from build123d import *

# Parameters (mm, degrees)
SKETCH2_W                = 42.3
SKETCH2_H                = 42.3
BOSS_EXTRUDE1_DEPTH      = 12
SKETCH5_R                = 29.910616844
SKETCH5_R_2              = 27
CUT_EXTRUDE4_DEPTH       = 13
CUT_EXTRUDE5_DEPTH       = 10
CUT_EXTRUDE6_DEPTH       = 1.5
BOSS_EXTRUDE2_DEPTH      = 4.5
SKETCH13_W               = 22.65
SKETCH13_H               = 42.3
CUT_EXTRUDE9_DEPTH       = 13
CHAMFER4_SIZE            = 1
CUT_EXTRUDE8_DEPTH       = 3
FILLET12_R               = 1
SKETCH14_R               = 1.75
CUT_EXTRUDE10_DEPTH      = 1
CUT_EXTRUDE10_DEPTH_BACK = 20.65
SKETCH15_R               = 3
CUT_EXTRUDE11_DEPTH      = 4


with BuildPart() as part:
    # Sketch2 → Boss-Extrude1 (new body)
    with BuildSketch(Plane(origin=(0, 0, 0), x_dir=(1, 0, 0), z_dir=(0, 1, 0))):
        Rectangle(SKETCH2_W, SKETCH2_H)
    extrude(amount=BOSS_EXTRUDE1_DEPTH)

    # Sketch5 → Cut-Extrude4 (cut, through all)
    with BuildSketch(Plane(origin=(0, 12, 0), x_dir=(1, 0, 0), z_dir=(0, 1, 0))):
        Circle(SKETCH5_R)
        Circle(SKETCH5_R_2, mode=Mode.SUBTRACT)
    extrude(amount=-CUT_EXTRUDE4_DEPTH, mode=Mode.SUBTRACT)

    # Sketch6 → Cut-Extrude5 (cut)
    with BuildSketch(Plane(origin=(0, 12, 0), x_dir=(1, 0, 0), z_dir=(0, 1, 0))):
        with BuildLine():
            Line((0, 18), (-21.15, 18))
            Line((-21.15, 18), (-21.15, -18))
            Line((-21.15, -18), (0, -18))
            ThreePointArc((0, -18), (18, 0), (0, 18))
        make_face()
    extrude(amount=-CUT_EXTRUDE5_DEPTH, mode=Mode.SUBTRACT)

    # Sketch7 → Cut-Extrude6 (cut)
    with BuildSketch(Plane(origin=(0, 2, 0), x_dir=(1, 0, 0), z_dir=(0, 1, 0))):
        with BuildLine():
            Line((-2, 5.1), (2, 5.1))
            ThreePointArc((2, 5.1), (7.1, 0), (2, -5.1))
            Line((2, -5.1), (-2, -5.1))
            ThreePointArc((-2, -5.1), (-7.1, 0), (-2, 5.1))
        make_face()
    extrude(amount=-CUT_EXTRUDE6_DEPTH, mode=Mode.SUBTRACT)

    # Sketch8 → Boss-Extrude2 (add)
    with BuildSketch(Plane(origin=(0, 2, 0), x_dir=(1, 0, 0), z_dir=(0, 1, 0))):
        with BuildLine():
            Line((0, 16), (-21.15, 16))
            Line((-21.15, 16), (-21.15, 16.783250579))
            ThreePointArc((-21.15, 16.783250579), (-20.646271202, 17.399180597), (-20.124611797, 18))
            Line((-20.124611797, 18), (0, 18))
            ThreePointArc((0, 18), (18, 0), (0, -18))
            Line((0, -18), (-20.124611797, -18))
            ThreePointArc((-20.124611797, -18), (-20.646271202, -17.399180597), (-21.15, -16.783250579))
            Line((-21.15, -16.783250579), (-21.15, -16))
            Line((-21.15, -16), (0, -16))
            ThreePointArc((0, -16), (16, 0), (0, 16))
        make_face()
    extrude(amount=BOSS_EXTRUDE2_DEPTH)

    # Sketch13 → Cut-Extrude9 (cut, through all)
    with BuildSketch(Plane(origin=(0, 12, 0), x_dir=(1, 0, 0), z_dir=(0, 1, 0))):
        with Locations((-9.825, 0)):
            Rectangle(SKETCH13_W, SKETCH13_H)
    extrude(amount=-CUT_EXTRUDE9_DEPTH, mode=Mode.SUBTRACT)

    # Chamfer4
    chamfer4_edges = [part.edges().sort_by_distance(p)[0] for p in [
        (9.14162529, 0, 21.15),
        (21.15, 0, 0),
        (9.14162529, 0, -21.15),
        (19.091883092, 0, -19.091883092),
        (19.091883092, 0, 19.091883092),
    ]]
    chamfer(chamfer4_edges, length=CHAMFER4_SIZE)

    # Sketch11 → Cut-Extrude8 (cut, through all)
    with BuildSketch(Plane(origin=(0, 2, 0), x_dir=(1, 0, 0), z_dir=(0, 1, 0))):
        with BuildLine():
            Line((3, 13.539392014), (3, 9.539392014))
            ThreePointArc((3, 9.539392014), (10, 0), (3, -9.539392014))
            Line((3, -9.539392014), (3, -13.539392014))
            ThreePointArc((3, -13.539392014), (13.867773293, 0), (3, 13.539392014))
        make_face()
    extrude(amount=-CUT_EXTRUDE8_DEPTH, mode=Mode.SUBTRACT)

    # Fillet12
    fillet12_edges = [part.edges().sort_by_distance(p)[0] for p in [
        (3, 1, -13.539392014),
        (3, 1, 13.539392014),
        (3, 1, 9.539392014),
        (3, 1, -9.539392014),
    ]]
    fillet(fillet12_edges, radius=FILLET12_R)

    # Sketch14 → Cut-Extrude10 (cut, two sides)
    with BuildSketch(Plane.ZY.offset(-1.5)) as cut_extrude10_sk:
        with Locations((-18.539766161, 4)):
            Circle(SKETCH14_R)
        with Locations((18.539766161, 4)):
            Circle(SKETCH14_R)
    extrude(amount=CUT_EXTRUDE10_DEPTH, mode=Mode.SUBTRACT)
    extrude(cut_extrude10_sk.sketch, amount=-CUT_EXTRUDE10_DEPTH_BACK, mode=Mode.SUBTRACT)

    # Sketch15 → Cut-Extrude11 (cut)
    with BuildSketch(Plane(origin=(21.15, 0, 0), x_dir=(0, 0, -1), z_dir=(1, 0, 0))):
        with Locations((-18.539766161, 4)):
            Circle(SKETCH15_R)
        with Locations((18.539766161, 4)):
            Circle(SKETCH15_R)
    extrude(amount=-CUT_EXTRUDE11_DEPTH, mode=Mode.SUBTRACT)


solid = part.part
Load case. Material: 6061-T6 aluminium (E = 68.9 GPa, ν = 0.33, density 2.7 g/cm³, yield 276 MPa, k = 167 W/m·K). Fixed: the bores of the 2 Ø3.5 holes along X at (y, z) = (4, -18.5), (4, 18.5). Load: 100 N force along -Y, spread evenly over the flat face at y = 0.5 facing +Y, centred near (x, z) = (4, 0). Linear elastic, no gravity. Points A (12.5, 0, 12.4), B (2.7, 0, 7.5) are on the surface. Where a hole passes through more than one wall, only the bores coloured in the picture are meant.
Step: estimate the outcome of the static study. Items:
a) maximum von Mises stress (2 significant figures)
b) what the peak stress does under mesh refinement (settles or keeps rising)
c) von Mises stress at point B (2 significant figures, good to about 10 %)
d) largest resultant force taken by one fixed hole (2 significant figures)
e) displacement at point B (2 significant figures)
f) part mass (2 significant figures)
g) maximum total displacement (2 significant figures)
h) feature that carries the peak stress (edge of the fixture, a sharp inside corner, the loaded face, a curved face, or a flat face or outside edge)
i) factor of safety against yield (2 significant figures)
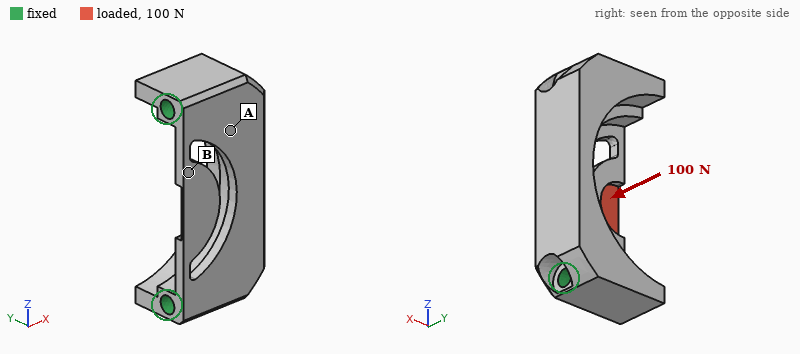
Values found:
240 MPa
settles
51 MPa
100 N
0.075 mm
13 g
0.20 mm
a curved face
1.1
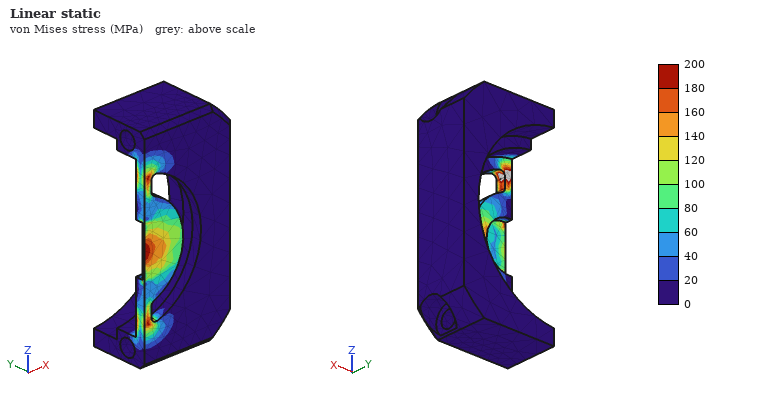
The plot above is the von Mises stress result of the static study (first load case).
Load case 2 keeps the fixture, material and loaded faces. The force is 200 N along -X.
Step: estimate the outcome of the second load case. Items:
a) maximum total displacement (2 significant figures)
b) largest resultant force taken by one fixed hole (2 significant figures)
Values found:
78 µm
140 N
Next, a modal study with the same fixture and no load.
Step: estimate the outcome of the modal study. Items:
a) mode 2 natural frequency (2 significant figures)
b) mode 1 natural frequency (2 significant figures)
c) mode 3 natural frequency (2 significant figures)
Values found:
15 kHz
5200 Hz
17 kHz
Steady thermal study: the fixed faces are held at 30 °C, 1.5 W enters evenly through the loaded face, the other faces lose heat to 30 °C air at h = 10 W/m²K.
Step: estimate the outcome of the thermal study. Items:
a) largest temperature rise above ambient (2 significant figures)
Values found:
14 K
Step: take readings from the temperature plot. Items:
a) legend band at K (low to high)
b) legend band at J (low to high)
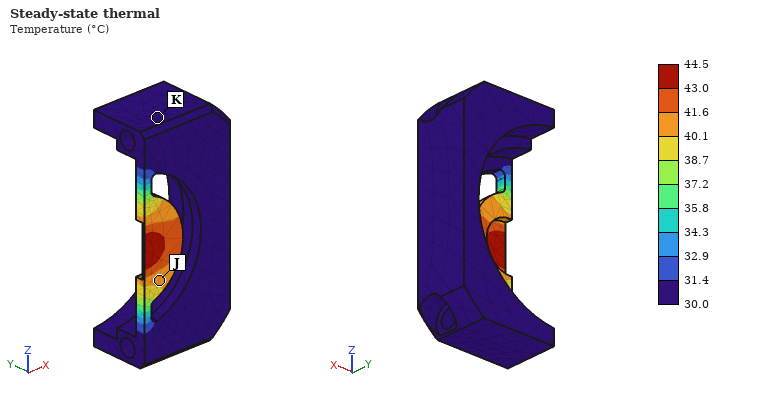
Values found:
30.0 to 31.4 °C
40.1 to 41.6 °C
